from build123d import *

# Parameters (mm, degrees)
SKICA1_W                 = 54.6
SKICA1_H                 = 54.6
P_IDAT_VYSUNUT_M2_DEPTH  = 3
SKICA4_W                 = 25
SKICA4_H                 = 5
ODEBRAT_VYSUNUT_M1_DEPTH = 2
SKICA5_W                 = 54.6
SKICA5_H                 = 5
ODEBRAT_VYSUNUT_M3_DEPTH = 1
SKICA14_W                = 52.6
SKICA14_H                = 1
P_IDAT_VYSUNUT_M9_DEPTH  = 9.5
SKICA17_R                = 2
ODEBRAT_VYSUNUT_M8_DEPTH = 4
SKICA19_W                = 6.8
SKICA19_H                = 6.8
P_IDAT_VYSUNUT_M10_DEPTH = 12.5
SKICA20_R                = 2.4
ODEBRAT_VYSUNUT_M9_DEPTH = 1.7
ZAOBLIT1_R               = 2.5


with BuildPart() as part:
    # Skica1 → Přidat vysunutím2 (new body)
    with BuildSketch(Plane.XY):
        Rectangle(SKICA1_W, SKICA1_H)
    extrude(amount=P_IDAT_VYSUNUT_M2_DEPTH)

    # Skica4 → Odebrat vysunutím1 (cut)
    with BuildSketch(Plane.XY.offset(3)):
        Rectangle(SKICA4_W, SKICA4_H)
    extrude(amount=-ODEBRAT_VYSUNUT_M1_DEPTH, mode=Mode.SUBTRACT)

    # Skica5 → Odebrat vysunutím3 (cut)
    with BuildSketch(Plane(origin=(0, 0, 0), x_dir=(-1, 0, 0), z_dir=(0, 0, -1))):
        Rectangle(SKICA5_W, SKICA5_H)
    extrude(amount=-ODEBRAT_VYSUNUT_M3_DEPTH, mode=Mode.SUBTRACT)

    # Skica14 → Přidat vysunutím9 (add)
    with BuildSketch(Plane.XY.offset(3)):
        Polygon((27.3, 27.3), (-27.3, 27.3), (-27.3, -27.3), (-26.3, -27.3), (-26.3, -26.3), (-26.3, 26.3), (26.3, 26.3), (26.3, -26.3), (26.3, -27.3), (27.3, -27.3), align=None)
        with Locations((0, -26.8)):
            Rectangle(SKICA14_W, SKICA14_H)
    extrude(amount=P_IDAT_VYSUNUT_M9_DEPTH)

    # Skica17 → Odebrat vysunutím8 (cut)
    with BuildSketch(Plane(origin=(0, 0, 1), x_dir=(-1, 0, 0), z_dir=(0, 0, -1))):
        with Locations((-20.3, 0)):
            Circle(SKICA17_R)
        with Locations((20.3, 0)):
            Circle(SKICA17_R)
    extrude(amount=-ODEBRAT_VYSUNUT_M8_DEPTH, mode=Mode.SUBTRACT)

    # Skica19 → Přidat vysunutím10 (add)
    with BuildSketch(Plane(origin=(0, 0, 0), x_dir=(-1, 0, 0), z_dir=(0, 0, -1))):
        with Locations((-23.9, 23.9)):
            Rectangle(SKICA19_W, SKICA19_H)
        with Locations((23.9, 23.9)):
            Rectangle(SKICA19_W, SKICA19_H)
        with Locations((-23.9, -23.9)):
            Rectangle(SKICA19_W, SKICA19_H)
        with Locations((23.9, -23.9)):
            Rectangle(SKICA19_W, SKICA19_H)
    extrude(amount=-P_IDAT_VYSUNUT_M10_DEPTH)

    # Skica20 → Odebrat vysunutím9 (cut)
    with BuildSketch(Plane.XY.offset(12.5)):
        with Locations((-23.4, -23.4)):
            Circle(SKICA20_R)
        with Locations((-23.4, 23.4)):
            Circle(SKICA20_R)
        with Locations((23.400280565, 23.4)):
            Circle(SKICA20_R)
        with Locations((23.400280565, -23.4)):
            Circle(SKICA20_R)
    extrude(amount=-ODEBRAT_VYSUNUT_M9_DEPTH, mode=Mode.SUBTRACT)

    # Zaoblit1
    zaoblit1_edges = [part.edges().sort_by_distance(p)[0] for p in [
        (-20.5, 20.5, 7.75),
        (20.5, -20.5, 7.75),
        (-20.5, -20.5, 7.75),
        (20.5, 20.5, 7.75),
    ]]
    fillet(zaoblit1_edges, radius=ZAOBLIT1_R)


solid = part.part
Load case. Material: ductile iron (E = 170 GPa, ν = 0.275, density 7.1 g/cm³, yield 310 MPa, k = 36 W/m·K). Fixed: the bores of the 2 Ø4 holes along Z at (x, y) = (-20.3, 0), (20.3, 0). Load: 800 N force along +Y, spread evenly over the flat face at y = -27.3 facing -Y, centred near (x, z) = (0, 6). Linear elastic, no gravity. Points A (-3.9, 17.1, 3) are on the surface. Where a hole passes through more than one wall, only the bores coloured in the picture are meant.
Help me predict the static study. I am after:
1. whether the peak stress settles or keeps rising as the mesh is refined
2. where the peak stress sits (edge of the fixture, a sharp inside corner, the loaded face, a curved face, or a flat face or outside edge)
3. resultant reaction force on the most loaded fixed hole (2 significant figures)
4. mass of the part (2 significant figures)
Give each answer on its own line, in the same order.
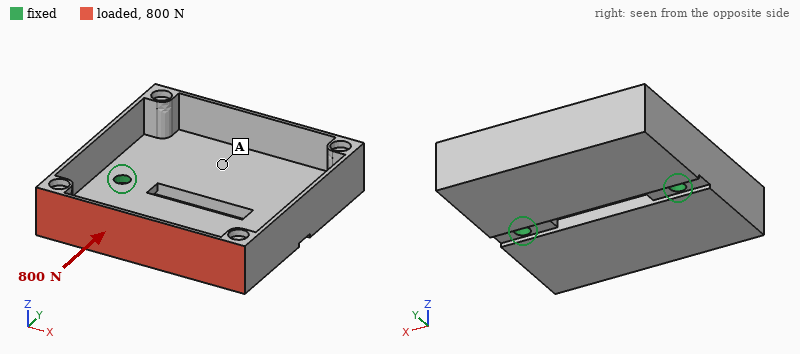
keeps rising
edge of the fixture
420 N
82 g
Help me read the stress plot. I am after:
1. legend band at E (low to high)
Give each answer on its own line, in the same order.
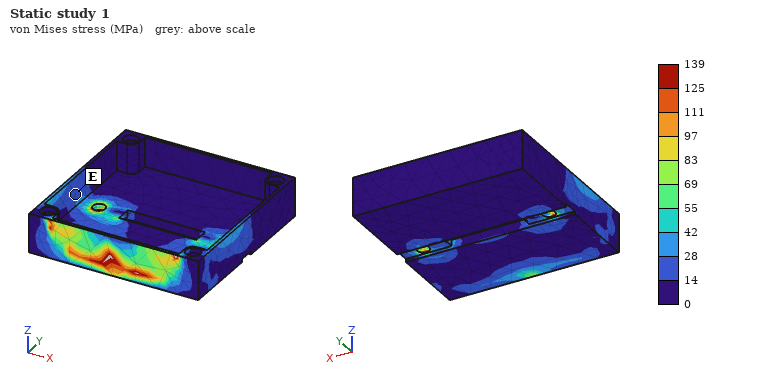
14 to 28 MPa
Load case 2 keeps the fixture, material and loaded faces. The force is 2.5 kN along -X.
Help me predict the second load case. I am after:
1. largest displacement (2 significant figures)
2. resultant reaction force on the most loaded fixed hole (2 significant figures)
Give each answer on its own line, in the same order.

0.12 mm
2.0 kN
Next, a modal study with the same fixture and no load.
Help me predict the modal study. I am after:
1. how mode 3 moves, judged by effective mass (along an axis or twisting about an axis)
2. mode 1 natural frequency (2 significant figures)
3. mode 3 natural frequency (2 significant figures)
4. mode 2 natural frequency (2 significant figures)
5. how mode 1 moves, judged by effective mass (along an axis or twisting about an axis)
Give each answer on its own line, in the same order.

along Z
1700 Hz
3800 Hz
2900 Hz
twisting about X
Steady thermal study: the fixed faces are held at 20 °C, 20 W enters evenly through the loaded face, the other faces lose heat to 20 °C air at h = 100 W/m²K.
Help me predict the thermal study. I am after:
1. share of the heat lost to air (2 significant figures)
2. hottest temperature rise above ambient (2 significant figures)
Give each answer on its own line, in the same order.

73 %
77 K
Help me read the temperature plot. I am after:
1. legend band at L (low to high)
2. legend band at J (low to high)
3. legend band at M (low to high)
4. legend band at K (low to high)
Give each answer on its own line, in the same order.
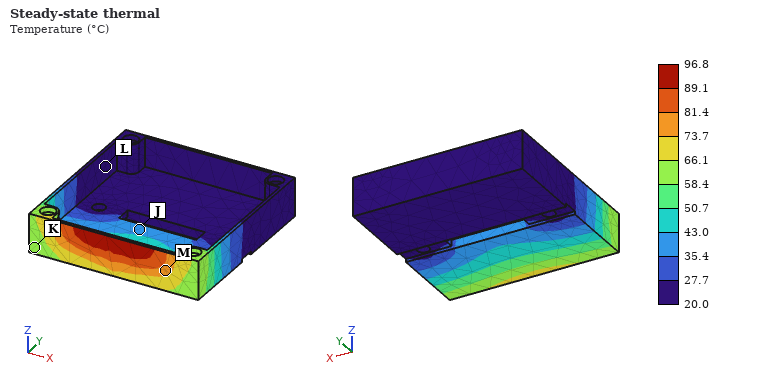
20.0 to 27.7 °C
35.4 to 43.0 °C
73.7 to 81.4 °C
58.4 to 66.1 °C
